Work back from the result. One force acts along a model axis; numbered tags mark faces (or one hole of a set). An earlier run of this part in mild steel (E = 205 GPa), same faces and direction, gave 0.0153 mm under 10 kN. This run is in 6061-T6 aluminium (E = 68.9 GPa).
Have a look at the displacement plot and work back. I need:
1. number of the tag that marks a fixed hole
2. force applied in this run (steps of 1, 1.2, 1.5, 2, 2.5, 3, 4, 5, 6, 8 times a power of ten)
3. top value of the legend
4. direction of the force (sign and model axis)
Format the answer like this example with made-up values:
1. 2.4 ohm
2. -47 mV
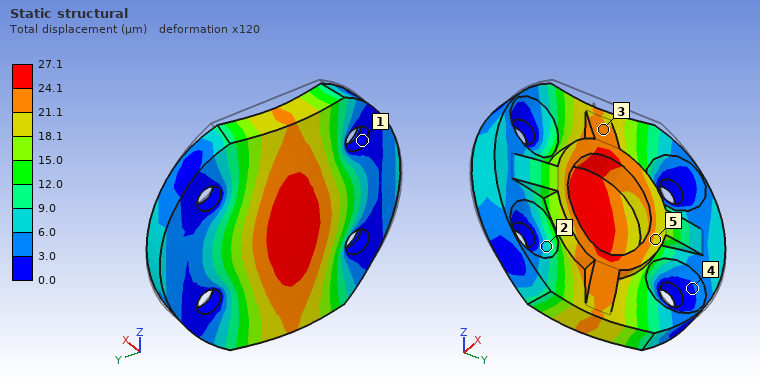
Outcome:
1. 1
2. 6 kN
3. 27.1 µm
4. -X
